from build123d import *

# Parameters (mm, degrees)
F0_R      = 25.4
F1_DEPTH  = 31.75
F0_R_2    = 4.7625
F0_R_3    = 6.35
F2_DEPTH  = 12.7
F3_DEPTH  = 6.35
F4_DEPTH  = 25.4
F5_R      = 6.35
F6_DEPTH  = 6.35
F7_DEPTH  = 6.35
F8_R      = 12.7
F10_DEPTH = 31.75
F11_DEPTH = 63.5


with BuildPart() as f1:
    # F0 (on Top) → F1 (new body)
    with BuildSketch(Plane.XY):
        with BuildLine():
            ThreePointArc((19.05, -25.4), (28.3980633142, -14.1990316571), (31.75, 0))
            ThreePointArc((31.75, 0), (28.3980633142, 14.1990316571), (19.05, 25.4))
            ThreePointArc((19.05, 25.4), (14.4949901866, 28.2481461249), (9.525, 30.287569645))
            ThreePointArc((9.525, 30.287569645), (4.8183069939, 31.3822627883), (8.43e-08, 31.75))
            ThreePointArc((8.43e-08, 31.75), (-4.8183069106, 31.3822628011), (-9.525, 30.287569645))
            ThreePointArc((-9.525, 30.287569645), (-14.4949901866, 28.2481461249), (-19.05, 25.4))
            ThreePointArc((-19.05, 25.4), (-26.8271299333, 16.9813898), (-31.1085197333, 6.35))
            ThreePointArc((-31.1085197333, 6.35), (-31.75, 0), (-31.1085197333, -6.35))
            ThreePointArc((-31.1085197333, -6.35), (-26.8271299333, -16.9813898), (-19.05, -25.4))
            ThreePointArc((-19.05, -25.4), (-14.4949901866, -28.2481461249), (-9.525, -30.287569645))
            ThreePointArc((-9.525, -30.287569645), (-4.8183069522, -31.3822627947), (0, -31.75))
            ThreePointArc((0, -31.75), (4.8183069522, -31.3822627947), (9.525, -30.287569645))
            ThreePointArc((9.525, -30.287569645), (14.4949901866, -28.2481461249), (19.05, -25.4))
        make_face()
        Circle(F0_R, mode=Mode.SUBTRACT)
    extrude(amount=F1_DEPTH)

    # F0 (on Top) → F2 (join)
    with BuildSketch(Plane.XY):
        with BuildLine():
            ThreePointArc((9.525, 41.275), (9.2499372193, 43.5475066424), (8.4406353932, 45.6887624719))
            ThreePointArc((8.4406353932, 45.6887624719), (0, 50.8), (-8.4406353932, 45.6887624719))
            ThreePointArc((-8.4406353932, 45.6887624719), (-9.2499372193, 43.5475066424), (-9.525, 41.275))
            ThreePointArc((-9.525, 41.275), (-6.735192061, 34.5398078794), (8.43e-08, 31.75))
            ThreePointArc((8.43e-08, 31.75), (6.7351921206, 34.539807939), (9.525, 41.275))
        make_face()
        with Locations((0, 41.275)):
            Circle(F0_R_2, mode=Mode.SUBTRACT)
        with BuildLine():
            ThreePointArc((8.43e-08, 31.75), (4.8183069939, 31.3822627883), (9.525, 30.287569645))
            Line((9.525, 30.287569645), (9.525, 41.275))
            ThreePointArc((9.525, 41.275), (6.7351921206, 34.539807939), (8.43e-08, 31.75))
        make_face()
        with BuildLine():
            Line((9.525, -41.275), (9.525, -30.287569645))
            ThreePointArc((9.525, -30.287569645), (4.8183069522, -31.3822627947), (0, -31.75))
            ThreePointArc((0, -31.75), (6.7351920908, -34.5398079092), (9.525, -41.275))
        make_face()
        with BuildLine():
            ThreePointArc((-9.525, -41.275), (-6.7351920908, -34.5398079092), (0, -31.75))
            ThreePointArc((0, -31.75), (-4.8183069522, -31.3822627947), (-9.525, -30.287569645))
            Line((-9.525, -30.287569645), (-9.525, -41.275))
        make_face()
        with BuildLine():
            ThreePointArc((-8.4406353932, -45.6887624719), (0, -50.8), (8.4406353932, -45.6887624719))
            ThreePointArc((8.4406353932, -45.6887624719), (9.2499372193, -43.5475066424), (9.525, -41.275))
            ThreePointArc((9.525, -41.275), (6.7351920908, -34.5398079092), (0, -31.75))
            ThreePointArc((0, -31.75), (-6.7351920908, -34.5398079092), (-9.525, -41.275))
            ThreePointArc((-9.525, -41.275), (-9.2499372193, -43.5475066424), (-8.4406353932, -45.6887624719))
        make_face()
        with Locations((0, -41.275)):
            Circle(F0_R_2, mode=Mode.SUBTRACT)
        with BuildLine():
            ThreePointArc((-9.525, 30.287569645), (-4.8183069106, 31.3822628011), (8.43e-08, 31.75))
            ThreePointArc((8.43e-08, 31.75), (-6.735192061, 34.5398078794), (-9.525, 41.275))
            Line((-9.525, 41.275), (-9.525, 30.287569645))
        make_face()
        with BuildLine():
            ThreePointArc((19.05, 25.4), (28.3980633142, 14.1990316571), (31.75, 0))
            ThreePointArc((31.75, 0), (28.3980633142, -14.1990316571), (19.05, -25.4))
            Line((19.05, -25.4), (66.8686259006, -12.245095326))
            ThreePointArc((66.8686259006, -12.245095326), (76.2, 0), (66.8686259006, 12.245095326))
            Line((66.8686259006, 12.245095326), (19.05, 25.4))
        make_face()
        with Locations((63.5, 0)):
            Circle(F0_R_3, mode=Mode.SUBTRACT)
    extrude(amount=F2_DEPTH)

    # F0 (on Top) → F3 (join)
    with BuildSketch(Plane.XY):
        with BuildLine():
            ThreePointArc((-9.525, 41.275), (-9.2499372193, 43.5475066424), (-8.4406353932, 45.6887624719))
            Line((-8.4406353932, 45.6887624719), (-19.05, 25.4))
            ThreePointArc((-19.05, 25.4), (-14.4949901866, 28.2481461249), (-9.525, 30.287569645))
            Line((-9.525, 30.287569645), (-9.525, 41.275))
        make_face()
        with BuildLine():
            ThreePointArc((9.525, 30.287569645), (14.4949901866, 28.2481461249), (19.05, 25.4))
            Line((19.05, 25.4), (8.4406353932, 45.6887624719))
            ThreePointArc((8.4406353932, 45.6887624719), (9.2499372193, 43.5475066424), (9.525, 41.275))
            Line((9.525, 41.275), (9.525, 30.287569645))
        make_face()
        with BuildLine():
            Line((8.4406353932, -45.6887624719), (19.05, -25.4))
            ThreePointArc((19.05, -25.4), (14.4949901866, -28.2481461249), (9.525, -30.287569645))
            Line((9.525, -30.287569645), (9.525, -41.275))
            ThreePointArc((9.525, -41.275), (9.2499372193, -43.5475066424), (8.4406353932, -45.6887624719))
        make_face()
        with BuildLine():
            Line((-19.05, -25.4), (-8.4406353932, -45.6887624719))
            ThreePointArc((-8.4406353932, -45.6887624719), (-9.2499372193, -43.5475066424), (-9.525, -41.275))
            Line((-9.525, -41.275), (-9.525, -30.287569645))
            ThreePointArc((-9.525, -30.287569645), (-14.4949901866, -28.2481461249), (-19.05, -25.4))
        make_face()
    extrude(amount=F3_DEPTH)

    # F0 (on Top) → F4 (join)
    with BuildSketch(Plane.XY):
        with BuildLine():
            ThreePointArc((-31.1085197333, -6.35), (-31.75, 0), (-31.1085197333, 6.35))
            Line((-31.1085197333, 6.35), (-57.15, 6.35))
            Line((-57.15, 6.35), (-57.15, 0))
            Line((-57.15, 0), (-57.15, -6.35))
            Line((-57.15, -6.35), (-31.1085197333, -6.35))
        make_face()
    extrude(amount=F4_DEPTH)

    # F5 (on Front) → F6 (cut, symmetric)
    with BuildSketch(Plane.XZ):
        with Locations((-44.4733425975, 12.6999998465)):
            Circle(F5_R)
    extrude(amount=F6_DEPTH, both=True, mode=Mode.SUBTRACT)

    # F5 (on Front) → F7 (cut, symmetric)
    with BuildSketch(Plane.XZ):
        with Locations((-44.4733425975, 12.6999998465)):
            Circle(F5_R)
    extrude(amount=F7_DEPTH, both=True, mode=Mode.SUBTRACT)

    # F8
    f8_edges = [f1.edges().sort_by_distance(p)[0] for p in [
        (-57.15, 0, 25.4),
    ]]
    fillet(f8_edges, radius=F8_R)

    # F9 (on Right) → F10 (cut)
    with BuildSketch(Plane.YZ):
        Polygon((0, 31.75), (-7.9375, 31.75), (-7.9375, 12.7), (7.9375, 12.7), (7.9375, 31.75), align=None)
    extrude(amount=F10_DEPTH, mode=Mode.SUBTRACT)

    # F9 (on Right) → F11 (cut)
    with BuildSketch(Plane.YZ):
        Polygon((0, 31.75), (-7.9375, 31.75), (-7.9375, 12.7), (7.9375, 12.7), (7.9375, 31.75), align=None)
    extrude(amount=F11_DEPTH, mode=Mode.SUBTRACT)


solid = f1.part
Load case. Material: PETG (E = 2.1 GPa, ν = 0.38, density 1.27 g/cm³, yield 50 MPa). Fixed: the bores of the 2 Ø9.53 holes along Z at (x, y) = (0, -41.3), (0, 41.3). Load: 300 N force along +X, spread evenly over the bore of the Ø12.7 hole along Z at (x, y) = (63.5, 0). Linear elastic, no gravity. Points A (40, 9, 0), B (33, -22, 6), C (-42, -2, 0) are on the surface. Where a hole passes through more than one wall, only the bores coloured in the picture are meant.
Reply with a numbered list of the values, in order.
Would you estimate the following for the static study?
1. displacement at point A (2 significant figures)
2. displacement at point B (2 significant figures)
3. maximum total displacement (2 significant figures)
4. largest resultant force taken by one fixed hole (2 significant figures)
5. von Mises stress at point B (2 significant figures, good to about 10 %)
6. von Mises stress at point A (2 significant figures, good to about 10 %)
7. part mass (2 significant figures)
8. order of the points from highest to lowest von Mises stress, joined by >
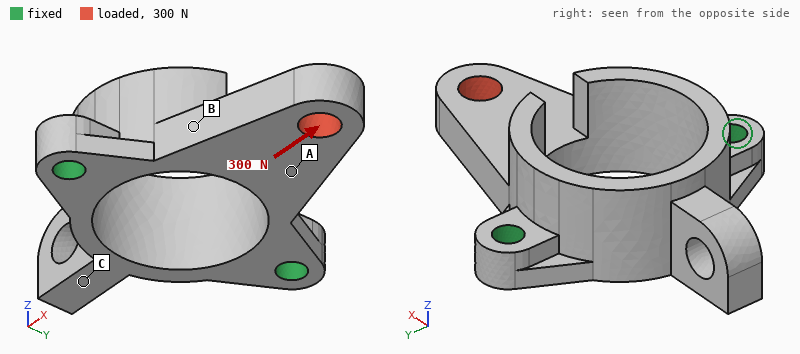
1. 45 µm
2. 32 µm
3. 76 µm
4. 170 N
5. 1.1 MPa
6. 0.61 MPa
7. 84 g
8. B > A > C
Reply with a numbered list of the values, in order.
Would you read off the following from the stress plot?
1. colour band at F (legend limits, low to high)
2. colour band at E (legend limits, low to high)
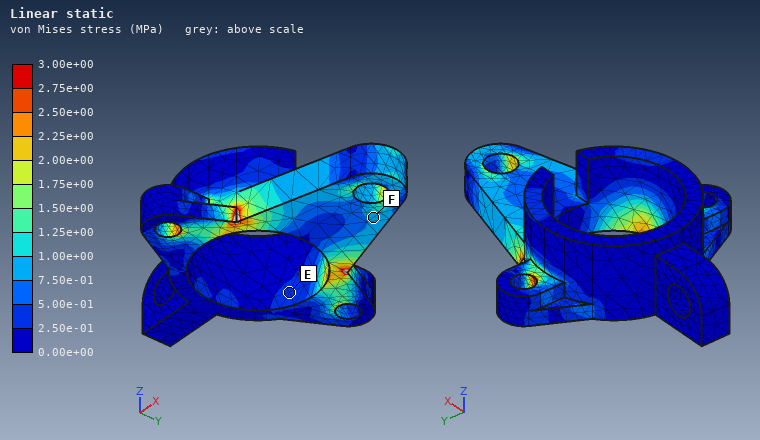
1. 7.50e-01 to 1.00e+00 MPa
2. 2.50e-01 to 5.00e-01 MPa
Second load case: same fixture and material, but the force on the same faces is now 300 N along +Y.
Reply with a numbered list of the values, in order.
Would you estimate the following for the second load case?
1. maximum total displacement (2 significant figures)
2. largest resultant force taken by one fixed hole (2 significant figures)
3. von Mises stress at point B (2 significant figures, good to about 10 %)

1. 0.25 mm
2. 320 N
3. 3.3 MPa
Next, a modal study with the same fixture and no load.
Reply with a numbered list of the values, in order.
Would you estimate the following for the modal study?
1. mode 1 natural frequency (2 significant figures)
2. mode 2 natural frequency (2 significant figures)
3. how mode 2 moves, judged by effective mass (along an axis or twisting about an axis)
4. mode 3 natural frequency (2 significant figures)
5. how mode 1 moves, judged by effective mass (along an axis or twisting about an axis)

1. 480 Hz
2. 840 Hz
3. along Z
4. 1600 Hz
5. along Z
